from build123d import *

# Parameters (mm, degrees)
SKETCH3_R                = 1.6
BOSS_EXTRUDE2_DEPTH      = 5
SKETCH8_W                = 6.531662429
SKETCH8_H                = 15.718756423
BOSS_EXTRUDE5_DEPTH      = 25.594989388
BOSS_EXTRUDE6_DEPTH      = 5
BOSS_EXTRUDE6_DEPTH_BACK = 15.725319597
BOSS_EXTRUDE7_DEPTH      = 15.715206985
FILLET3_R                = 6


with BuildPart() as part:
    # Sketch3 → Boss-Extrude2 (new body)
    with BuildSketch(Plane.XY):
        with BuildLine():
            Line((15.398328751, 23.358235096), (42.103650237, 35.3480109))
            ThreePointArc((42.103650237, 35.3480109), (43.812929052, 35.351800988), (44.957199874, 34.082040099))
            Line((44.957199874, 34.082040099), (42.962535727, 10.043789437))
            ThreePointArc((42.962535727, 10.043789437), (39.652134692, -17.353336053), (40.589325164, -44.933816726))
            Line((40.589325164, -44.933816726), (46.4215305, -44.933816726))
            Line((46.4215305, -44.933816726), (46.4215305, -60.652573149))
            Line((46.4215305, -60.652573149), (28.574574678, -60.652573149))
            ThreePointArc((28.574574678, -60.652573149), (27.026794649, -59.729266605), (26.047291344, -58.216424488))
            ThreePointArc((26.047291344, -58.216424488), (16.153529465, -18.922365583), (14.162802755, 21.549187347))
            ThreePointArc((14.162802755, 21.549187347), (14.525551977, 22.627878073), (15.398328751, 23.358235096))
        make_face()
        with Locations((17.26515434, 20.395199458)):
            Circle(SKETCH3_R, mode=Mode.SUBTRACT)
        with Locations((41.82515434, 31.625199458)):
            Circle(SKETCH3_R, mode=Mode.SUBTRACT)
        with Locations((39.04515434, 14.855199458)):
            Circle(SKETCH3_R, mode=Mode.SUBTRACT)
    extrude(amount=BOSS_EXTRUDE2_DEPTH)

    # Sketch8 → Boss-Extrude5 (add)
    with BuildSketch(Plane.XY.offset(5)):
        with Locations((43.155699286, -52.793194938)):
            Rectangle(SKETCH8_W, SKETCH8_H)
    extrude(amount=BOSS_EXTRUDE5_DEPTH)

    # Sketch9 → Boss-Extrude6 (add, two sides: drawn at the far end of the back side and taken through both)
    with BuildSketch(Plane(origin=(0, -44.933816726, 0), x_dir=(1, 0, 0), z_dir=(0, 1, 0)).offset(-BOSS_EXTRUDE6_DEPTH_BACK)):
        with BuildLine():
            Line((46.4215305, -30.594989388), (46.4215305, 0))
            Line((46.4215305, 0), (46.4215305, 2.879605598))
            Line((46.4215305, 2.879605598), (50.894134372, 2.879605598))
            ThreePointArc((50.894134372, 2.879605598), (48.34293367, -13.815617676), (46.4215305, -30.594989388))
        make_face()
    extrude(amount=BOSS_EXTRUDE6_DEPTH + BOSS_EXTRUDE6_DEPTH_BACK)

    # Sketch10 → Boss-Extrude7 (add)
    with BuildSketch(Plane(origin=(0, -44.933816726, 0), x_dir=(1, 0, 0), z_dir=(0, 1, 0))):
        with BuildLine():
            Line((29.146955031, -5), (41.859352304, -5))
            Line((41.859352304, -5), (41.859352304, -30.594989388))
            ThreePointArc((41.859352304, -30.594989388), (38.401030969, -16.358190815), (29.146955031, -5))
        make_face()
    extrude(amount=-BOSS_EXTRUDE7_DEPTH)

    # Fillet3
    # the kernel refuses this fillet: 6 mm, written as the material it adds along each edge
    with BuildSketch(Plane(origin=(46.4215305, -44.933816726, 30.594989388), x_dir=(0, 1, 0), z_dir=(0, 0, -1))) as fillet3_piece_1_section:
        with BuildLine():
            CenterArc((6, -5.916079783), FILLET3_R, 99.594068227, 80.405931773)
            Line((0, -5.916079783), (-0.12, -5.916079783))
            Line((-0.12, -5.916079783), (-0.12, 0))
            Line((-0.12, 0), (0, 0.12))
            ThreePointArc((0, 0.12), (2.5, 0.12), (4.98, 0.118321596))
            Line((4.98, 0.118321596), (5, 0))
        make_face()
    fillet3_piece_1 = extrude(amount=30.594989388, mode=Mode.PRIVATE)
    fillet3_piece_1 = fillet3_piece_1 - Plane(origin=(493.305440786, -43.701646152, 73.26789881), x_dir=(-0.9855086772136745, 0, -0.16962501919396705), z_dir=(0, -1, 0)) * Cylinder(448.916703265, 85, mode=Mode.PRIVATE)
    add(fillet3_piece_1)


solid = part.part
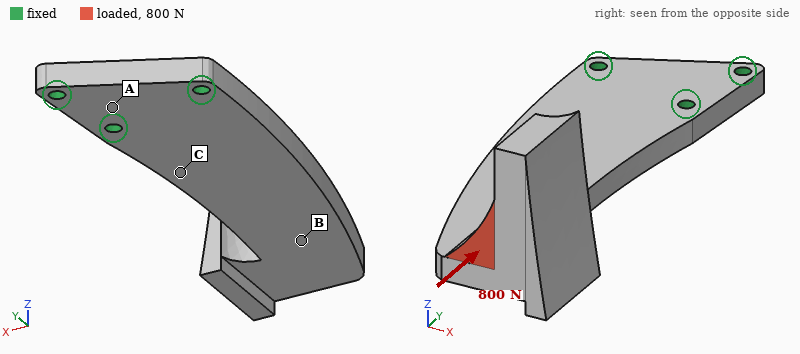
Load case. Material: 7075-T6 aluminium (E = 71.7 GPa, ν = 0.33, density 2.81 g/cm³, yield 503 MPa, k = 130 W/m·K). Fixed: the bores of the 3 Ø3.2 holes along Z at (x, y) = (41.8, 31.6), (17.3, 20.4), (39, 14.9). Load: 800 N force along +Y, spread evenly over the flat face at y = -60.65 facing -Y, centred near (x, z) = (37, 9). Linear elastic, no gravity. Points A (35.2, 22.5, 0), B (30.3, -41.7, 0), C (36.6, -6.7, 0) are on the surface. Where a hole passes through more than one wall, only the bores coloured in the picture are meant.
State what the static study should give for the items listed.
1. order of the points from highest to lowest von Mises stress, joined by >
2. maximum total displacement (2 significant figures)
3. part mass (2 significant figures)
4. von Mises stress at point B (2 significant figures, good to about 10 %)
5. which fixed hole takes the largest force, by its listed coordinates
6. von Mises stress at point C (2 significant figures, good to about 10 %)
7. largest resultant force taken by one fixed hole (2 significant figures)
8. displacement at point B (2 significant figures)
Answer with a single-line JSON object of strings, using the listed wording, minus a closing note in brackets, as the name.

{"order of the points from highest to lowest von Mises stress, joined by >": "B > C > A", "maximum total displacement": "1.1 mm", "part mass": "46 g", "von Mises stress at point B": "56 MPa", "which fixed hole takes the largest force, by its listed coordinates": "(39, 14.9)", "von Mises stress at point C": "38 MPa", "largest resultant force taken by one fixed hole": "660 N", "displacement at point B": "0.50 mm"}
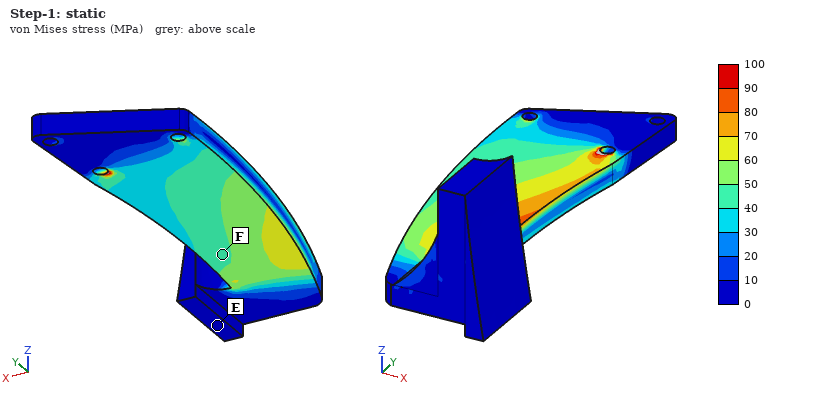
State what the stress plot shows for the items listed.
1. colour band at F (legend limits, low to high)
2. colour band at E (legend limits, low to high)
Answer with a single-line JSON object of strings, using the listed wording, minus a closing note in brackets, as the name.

{"colour band at F": "40 to 50 MPa", "colour band at E": "0 to 10 MPa"}
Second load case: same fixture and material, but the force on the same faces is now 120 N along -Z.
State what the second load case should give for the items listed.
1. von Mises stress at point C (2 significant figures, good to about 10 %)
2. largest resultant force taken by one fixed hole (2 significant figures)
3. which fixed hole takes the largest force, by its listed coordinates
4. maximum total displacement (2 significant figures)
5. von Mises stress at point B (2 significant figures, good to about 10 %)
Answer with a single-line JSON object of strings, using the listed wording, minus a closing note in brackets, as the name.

{"von Mises stress at point C": "65 MPa", "largest resultant force taken by one fixed hole": "320 N", "which fixed hole takes the largest force, by its listed coordinates": "(39, 14.9)", "maximum total displacement": "1.1 mm", "von Mises stress at point B": "29 MPa"}
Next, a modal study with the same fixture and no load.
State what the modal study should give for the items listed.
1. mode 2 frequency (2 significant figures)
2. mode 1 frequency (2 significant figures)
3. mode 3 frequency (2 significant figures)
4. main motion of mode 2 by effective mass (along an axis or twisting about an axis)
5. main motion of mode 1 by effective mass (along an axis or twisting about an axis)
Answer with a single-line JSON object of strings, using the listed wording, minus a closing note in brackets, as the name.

{"mode 2 frequency": "1400 Hz", "mode 1 frequency": "430 Hz", "mode 3 frequency": "2300 Hz", "main motion of mode 2 by effective mass": "along X", "main motion of mode 1 by effective mass": "along Z"}
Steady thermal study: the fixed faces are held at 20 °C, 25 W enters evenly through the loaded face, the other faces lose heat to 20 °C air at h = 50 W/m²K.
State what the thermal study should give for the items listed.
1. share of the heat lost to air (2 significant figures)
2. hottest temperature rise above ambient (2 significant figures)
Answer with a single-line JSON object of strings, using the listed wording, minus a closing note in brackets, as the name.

{"share of the heat lost to air": "52 %", "hottest temperature rise above ambient": "80 K"}
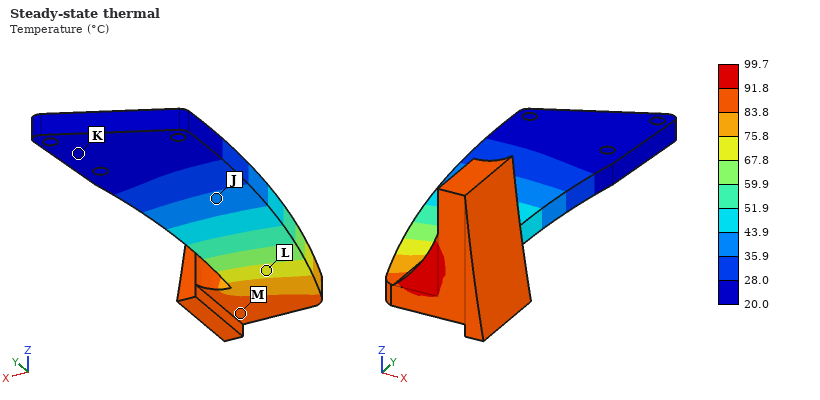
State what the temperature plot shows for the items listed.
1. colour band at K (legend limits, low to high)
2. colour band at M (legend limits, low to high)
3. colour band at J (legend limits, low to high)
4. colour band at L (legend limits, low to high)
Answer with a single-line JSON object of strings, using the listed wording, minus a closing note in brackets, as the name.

{"colour band at K": "20.0 to 28.0 °C", "colour band at M": "83.8 to 91.8 °C", "colour band at J": "35.9 to 43.9 °C", "colour band at L": "67.8 to 75.8 °C"}
